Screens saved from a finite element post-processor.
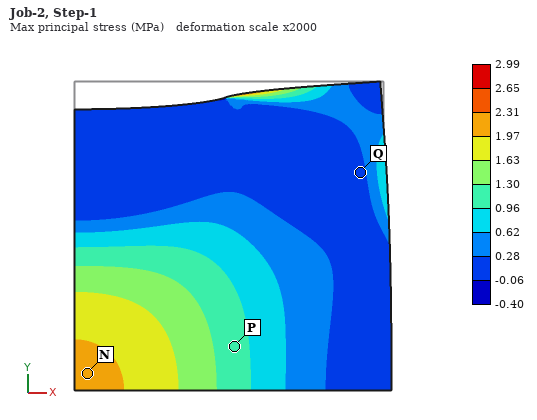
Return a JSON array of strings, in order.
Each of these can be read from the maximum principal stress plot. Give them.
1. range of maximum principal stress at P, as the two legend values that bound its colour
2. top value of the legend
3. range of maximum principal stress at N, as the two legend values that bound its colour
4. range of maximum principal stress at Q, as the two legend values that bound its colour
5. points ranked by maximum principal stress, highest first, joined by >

["0.96 to 1.30 MPa", "2.99 MPa", "1.97 to 2.31 MPa", "-0.06 to 0.28 MPa", "N > P > Q"]
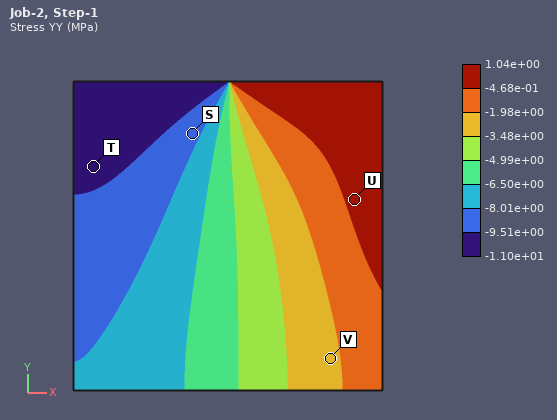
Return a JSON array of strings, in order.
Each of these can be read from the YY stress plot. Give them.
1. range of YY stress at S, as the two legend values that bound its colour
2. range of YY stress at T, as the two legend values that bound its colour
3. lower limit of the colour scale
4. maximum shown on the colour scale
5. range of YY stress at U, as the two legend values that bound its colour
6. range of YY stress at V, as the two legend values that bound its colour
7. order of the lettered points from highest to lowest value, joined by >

["-9.51e+00 to -8.01e+00 MPa", "-1.10e+01 to -9.51e+00 MPa", "-1.10e+01 MPa", "1.04e+00 MPa", "-4.68e-01 to 1.04e+00 MPa", "-3.48e+00 to -1.98e+00 MPa", "U > V > S > T"]
